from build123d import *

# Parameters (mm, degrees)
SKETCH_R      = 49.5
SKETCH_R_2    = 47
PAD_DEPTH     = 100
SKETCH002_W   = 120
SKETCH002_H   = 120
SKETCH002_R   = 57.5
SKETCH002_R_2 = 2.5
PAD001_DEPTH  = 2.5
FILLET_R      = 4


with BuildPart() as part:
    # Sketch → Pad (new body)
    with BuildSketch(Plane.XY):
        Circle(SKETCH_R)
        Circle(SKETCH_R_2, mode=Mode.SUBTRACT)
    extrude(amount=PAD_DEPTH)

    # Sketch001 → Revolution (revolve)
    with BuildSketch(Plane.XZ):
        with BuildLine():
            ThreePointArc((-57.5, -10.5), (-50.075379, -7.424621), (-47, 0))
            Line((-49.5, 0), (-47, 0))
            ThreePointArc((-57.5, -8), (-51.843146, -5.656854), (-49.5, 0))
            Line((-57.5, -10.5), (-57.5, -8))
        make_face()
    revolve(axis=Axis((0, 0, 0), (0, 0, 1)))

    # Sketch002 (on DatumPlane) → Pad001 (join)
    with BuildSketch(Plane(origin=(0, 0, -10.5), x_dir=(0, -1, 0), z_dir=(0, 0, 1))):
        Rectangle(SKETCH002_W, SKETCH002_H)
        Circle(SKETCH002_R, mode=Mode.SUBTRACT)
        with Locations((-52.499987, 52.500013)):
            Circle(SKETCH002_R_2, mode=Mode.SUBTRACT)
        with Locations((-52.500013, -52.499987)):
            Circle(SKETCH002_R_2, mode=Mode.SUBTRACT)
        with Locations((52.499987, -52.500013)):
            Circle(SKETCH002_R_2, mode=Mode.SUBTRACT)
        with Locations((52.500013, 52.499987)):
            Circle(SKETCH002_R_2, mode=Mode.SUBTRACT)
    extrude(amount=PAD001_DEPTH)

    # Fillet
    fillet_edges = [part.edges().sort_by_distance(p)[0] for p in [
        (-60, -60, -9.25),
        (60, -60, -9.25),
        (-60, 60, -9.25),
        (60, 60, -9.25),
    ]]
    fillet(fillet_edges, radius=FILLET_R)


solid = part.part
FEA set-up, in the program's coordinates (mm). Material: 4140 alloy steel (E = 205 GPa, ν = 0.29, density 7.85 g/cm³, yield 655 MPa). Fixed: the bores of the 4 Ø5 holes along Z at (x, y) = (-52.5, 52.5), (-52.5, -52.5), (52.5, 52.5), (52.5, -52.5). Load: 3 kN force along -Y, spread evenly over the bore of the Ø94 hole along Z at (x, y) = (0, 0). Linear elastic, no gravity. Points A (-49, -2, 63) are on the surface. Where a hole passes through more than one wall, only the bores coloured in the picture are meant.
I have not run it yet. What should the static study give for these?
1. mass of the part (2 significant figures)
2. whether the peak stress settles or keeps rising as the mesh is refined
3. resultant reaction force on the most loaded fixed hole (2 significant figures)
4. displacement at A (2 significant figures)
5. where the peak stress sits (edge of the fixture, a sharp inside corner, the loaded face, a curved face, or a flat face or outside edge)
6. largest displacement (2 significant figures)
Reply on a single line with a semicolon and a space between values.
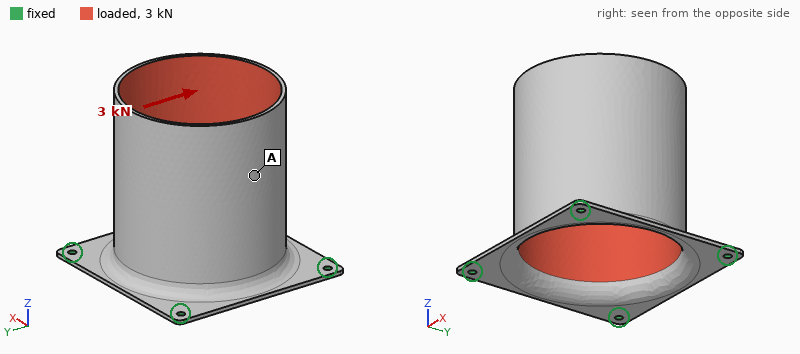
760 g; keeps rising; 1.5 kN; 0.29 mm; edge of the fixture; 0.48 mm
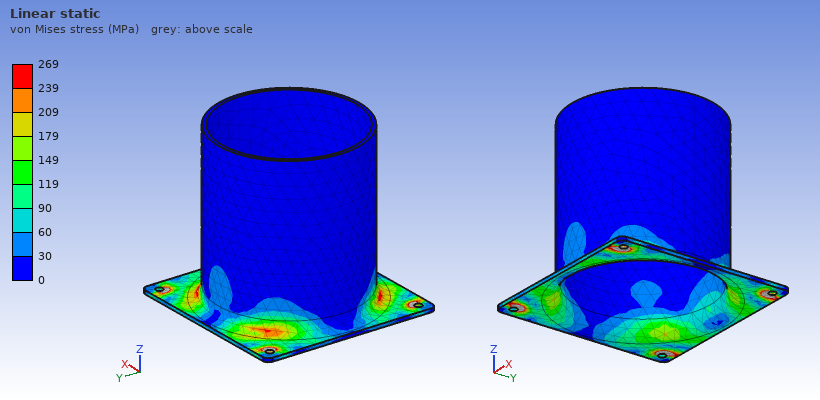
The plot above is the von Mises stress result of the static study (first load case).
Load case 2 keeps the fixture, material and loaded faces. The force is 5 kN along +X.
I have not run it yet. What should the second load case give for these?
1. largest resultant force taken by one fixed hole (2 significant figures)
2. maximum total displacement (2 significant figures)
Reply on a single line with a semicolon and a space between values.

2.5 kN; 0.81 mm
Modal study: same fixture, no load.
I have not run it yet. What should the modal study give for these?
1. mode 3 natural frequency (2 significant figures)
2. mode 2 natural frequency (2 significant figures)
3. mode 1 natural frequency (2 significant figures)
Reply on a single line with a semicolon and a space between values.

790 Hz; 570 Hz; 570 Hz
